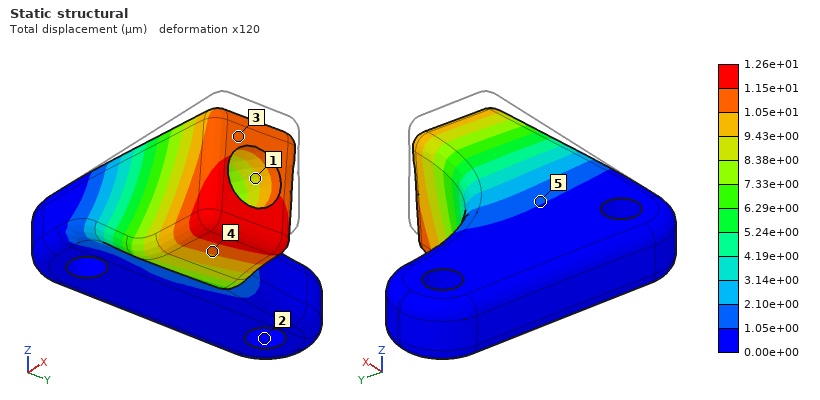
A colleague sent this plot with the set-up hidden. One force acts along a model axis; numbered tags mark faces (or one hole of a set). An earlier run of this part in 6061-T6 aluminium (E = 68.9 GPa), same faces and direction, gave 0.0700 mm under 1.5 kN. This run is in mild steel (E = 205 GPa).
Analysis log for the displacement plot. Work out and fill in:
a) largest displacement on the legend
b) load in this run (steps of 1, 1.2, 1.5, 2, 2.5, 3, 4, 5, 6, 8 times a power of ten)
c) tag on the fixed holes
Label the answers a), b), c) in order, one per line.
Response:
a) 1.26e+01 µm
b) 800 N
c) 2
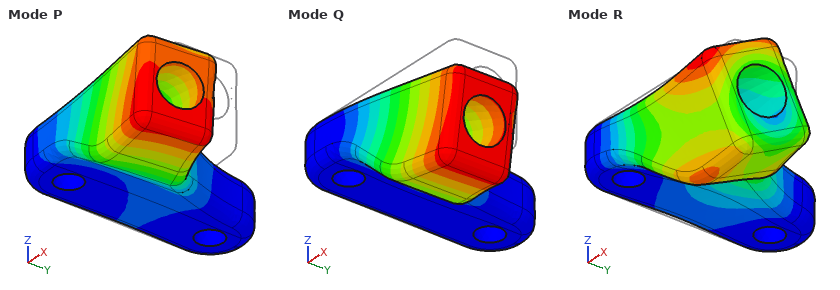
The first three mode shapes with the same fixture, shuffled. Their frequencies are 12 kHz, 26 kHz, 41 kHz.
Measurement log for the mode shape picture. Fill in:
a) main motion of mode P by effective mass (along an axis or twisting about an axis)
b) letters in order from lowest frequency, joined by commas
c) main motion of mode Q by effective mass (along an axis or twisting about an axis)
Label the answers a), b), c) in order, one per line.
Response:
a) along Y
b) Q, P, R
c) along Z
